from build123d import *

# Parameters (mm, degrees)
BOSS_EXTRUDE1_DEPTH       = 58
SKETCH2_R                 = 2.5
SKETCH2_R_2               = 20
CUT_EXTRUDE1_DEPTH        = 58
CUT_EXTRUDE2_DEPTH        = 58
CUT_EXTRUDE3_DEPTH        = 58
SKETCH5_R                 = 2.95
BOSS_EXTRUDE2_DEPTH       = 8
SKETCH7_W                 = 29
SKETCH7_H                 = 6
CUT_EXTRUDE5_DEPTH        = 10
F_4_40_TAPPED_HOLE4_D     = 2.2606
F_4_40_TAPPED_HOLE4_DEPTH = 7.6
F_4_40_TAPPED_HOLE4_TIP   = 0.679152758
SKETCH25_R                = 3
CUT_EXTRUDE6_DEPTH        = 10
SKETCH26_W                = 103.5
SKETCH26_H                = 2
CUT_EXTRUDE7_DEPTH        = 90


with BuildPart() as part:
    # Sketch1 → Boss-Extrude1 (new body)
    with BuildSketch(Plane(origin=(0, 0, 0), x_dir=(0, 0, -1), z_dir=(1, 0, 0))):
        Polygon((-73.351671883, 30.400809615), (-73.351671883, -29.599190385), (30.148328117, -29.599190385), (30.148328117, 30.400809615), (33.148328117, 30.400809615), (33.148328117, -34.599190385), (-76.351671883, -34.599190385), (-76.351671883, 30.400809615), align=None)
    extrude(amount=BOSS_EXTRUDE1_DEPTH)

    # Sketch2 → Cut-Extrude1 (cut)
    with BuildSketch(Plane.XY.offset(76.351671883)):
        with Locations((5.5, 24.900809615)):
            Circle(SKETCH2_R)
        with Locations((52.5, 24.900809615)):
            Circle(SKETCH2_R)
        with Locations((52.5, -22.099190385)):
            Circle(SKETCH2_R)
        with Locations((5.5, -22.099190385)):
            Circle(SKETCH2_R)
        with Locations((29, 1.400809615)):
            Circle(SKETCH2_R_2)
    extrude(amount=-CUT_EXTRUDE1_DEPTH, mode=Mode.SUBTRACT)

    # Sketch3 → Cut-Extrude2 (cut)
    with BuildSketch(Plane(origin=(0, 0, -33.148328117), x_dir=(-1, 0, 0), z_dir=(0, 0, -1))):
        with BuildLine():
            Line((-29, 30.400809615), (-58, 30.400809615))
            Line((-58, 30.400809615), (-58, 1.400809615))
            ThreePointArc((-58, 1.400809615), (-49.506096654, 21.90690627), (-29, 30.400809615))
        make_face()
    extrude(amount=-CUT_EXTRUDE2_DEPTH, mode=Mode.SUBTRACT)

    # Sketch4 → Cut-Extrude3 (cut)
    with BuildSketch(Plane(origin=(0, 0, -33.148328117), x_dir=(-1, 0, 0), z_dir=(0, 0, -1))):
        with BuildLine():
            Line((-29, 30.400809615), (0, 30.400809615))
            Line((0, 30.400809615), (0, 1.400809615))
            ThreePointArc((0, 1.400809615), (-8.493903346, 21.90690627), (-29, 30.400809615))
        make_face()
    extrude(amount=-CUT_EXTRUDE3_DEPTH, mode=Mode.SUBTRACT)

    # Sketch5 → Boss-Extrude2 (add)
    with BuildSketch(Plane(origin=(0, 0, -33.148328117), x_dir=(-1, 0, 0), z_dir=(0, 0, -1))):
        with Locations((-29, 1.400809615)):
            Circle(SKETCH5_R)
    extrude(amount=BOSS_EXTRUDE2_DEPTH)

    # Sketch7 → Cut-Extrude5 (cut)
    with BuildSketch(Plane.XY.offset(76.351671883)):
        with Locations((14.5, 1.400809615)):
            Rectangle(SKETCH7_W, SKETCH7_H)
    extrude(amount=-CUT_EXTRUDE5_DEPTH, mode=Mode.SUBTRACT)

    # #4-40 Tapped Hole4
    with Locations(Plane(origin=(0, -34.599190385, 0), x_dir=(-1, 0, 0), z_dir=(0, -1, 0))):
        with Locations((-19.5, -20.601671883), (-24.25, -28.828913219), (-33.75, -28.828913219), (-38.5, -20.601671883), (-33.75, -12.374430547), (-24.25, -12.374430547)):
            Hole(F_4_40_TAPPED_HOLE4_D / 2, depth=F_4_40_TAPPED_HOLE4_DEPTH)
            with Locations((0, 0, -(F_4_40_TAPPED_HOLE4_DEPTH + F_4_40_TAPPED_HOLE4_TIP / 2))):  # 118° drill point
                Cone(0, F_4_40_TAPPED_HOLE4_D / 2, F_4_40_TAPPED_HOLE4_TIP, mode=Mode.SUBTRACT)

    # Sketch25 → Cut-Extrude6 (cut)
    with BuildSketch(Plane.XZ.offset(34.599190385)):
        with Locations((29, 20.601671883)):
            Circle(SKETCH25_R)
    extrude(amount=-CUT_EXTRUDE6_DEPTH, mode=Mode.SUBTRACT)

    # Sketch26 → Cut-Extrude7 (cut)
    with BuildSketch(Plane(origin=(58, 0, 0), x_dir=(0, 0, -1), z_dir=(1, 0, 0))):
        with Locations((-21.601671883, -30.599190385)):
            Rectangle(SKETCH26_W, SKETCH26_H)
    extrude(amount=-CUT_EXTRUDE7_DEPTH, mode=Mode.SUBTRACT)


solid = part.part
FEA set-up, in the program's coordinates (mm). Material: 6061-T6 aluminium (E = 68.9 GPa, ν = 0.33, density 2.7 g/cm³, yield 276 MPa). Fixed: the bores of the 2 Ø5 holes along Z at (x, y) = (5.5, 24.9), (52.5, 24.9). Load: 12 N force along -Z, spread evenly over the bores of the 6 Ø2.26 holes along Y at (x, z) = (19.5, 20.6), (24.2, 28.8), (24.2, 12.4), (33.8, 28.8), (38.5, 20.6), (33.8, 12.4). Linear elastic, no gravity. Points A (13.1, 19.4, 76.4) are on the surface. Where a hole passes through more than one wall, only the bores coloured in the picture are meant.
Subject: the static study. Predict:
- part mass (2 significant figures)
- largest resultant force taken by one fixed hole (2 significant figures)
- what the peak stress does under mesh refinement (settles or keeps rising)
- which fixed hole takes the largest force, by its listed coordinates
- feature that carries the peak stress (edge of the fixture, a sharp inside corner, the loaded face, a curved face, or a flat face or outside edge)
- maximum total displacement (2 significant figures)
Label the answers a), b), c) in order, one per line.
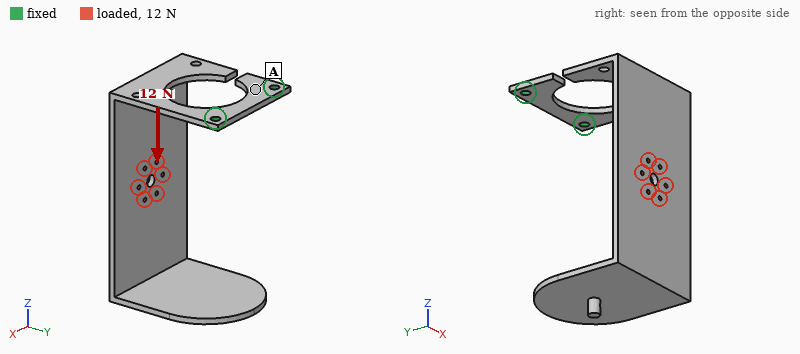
a) 96 g
b) 13 N
c) keeps rising
d) (52.5, 24.9)
e) edge of the fixture
f) 1.5 mm
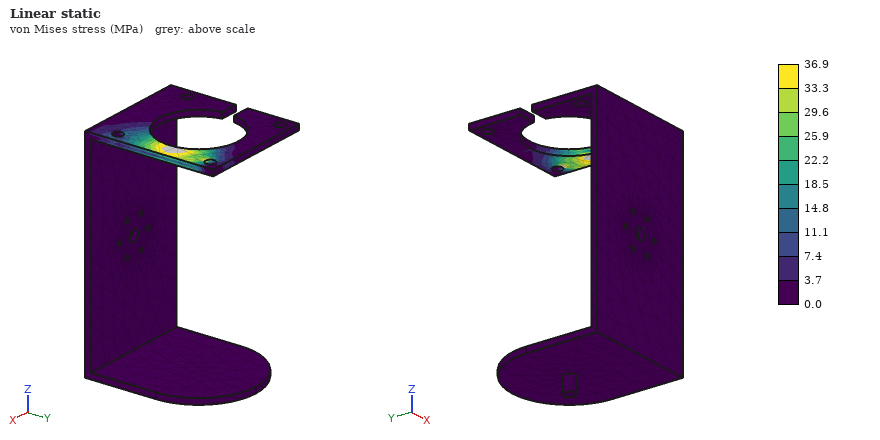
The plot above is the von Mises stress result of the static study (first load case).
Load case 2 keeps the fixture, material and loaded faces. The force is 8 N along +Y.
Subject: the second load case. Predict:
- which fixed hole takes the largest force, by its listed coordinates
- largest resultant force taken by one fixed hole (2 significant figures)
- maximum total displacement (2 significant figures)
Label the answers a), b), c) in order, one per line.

a) (52.5, 24.9)
b) 5.8 N
c) 1.5 mm
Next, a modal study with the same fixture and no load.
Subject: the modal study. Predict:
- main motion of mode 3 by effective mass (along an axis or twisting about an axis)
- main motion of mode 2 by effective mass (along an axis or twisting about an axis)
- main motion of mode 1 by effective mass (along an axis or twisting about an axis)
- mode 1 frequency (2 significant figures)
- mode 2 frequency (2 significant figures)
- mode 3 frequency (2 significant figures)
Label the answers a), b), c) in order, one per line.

a) along Z
b) along X
c) along Y
d) 38 Hz
e) 47 Hz
f) 170 Hz
